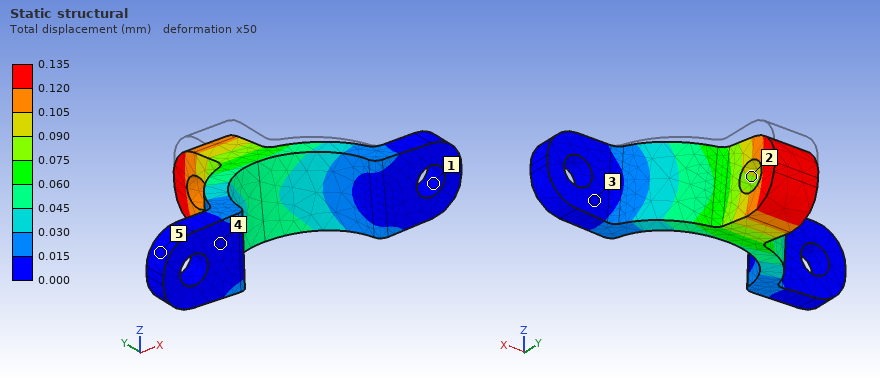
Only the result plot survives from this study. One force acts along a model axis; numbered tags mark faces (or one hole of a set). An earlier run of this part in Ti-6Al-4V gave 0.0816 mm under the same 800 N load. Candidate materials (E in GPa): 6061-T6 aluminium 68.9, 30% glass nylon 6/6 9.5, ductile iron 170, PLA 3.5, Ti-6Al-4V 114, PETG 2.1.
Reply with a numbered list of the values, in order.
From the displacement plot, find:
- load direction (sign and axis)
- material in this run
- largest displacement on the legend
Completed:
1. -Z
2. 6061-T6 aluminium
3. 0.135 mm
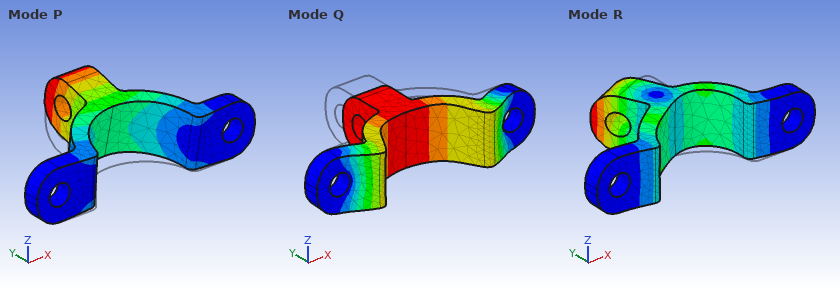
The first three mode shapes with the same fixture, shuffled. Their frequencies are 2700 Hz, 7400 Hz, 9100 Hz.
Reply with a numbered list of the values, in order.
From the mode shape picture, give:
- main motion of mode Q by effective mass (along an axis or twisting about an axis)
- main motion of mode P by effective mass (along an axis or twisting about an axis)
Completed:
1. along Y
2. along Z
